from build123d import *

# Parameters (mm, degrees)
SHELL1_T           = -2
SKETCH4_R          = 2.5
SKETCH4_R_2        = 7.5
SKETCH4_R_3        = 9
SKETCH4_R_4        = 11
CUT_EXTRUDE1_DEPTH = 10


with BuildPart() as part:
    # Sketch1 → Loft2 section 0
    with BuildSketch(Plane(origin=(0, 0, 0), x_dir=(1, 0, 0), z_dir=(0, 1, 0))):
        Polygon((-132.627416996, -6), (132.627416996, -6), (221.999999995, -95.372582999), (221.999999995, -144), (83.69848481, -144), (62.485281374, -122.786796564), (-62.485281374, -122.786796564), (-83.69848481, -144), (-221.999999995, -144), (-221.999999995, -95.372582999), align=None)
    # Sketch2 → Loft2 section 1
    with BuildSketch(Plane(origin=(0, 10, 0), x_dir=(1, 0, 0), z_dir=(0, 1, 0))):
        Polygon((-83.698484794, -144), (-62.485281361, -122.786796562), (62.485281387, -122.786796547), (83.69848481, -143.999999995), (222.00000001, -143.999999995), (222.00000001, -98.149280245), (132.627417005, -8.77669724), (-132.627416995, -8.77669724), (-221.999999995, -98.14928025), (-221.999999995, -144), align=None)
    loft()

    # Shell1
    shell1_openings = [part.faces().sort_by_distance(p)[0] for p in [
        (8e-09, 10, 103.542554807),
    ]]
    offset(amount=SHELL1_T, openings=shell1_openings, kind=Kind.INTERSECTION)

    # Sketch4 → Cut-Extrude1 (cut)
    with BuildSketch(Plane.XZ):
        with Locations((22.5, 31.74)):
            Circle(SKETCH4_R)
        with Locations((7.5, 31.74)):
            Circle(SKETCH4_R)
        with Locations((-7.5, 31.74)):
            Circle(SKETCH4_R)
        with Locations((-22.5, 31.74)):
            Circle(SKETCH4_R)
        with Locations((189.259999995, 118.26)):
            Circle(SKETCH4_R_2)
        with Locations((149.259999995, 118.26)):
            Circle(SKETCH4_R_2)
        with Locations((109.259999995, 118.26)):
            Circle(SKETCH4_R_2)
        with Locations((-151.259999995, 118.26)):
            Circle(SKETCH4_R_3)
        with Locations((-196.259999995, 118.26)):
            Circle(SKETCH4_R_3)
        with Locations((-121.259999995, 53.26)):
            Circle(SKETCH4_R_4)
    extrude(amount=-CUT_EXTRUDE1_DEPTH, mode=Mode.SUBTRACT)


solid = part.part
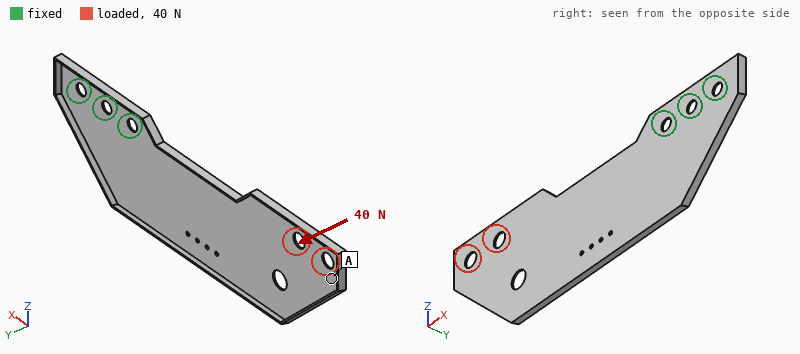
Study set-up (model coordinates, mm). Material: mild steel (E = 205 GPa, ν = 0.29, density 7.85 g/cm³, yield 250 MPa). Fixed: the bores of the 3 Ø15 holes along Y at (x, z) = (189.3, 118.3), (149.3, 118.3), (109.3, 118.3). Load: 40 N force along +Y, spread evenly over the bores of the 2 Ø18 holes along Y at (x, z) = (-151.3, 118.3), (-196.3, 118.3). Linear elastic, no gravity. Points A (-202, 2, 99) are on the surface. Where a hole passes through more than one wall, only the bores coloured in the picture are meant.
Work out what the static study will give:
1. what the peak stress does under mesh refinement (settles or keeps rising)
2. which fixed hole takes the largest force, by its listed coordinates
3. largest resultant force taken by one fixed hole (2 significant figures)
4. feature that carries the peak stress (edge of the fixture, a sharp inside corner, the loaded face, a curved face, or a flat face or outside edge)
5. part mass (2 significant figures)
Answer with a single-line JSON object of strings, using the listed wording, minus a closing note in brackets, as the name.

{"what the peak stress does under mesh refinement": "keeps rising", "which fixed hole takes the largest force, by its listed coordinates": "(109.3, 118.3)", "largest resultant force taken by one fixed hole": "360 N", "feature that carries the peak stress": "a sharp inside corner", "part mass": "900 g"}
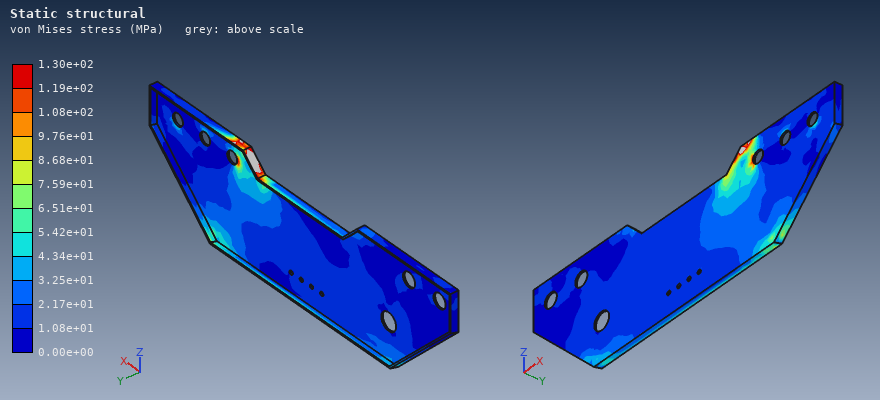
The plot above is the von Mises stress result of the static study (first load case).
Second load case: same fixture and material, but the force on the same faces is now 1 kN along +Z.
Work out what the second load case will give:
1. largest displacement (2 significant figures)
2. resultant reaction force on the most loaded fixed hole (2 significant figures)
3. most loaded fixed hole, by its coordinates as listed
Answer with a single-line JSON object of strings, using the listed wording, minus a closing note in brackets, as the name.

{"largest displacement": "0.32 mm", "resultant reaction force on the most loaded fixed hole": "4.5 kN", "most loaded fixed hole, by its coordinates as listed": "(109.3, 118.3)"}
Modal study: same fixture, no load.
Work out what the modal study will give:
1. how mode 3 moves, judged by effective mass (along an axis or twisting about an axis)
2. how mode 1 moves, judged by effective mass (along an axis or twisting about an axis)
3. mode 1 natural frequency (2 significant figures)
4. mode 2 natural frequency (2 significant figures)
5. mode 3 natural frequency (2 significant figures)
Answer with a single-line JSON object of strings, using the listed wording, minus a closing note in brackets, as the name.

{"how mode 3 moves, judged by effective mass": "along Y", "how mode 1 moves, judged by effective mass": "along Y", "mode 1 natural frequency": "32 Hz", "mode 2 natural frequency": "78 Hz", "mode 3 natural frequency": "190 Hz"}
